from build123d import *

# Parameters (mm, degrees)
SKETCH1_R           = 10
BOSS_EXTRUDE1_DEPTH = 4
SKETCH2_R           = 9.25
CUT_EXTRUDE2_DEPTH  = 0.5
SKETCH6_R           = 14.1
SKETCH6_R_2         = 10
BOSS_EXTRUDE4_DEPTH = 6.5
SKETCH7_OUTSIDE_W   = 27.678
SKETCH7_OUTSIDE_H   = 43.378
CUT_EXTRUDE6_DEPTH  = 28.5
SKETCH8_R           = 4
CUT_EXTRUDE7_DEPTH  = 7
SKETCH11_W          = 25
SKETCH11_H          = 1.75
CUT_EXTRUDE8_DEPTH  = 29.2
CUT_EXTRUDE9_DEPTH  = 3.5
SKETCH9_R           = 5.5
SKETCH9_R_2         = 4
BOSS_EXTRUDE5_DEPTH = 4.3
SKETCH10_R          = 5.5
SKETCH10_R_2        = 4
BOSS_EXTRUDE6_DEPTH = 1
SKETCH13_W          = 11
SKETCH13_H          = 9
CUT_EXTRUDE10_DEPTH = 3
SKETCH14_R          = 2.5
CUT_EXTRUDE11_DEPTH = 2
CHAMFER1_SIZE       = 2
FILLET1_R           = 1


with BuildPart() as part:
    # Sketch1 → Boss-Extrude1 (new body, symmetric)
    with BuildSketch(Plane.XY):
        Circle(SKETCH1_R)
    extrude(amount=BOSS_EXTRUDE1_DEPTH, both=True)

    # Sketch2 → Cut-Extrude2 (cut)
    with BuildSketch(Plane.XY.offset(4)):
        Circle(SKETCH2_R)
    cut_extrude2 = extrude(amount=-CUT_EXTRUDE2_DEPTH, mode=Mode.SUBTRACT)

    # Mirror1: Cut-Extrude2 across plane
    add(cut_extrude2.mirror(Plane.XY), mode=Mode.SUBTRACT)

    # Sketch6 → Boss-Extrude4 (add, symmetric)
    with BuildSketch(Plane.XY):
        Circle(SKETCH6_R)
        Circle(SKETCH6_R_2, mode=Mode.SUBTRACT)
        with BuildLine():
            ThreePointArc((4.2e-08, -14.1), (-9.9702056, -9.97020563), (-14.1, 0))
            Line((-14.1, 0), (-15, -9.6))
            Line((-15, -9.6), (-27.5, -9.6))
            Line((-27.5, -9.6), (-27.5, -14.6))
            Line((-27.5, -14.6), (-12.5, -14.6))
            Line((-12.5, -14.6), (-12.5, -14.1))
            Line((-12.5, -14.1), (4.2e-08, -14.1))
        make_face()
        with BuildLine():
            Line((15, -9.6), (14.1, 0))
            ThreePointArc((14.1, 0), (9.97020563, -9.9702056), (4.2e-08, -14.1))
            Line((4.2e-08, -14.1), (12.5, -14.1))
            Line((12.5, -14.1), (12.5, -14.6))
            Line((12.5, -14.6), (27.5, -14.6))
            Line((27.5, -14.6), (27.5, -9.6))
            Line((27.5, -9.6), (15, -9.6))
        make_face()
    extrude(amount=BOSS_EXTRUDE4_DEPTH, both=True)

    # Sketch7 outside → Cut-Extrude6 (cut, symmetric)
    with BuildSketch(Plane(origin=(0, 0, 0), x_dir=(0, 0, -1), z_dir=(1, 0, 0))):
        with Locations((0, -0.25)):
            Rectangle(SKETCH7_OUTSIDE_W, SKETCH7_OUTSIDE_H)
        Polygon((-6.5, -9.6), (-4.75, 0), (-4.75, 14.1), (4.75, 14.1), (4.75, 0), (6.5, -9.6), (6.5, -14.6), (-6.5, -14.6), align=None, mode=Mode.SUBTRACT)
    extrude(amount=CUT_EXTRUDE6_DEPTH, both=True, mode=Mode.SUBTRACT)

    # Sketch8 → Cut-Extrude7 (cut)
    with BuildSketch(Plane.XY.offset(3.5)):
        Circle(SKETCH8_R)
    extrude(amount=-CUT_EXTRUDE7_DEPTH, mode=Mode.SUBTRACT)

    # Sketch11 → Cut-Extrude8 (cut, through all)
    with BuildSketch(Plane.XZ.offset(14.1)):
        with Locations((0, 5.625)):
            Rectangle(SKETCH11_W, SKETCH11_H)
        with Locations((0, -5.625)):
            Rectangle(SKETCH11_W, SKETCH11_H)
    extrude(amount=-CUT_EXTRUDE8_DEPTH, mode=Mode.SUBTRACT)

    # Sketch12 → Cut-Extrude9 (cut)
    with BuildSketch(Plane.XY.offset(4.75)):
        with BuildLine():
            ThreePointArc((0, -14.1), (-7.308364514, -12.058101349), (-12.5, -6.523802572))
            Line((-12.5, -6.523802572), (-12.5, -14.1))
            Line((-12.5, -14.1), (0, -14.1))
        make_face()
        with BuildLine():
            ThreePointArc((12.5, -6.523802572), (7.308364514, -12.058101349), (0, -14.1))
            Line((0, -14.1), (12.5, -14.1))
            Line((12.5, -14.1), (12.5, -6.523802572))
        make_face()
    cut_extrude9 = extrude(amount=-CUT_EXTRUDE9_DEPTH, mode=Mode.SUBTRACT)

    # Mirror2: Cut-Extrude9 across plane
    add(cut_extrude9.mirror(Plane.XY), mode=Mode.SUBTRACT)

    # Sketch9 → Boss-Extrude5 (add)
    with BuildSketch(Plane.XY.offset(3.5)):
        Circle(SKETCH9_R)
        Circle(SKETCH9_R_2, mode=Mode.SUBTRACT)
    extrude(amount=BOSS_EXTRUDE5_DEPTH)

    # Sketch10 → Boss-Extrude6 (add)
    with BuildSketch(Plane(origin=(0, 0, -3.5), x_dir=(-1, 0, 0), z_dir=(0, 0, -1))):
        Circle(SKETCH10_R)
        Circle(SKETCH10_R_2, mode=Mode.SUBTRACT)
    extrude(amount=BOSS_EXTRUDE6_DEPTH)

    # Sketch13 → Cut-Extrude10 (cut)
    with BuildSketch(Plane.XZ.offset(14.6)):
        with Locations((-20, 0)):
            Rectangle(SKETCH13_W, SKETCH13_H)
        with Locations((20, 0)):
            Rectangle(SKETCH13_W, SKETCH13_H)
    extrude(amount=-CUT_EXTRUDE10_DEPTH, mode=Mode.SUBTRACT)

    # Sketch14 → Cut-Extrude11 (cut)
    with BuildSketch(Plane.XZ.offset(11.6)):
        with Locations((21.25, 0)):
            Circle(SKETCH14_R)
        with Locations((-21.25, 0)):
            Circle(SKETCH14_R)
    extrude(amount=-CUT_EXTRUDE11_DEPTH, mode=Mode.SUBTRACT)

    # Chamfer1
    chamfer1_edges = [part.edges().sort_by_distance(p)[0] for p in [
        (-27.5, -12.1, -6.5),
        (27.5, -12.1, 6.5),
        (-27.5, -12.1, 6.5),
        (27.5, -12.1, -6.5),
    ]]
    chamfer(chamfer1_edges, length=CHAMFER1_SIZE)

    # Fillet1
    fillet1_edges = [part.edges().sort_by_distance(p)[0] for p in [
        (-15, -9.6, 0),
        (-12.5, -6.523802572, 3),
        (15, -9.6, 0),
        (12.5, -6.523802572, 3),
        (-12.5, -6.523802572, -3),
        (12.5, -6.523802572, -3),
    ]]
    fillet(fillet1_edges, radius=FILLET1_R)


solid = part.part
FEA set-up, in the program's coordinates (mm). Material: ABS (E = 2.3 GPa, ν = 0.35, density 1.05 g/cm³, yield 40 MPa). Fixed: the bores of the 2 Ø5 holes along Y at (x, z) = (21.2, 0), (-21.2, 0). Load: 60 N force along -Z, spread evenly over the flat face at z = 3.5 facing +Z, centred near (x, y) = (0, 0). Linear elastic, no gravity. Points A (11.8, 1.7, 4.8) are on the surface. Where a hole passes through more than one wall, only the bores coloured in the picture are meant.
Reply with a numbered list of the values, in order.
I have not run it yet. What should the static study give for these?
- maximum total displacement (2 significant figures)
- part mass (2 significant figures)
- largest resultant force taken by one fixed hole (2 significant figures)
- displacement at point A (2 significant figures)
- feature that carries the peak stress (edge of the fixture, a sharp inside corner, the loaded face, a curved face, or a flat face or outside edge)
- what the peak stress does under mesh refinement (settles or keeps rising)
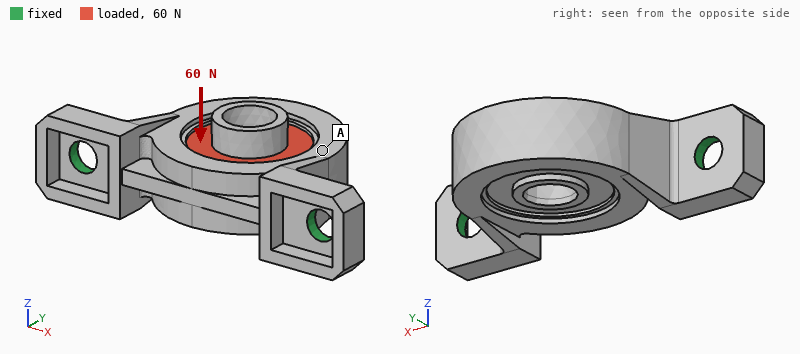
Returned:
1. 0.54 mm
2. 7.1 g
3. 30 N
4. 0.29 mm
5. edge of the fixture
6. keeps rising
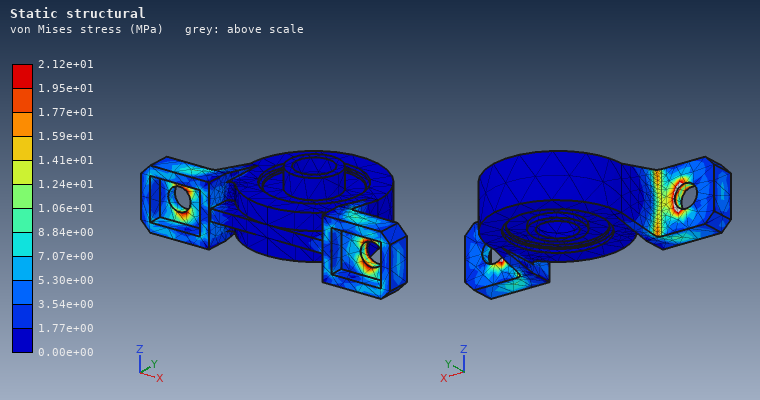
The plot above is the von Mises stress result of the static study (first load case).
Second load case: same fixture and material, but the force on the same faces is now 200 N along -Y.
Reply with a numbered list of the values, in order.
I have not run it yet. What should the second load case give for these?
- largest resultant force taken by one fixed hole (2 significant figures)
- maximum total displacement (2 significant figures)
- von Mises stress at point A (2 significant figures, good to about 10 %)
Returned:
1. 120 N
2. 0.61 mm
3. 2.9 MPa
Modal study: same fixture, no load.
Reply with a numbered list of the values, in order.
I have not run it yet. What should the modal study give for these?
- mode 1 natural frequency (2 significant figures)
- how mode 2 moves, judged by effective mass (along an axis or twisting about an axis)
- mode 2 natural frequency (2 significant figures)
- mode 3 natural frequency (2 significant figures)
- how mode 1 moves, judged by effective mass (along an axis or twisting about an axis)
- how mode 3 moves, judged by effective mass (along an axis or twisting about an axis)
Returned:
1. 890 Hz
2. along Y
3. 2800 Hz
4. 3300 Hz
5. along Z
6. along X
